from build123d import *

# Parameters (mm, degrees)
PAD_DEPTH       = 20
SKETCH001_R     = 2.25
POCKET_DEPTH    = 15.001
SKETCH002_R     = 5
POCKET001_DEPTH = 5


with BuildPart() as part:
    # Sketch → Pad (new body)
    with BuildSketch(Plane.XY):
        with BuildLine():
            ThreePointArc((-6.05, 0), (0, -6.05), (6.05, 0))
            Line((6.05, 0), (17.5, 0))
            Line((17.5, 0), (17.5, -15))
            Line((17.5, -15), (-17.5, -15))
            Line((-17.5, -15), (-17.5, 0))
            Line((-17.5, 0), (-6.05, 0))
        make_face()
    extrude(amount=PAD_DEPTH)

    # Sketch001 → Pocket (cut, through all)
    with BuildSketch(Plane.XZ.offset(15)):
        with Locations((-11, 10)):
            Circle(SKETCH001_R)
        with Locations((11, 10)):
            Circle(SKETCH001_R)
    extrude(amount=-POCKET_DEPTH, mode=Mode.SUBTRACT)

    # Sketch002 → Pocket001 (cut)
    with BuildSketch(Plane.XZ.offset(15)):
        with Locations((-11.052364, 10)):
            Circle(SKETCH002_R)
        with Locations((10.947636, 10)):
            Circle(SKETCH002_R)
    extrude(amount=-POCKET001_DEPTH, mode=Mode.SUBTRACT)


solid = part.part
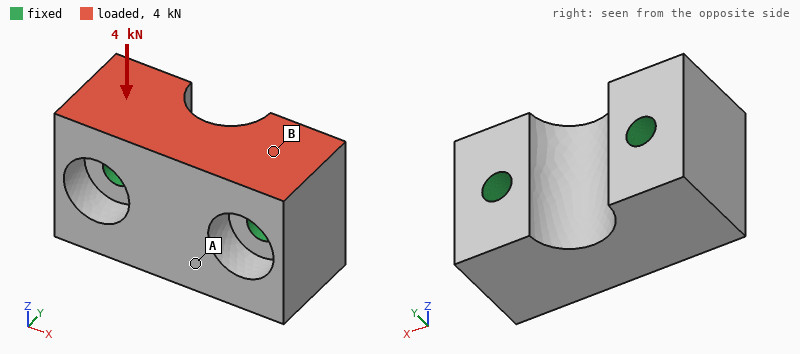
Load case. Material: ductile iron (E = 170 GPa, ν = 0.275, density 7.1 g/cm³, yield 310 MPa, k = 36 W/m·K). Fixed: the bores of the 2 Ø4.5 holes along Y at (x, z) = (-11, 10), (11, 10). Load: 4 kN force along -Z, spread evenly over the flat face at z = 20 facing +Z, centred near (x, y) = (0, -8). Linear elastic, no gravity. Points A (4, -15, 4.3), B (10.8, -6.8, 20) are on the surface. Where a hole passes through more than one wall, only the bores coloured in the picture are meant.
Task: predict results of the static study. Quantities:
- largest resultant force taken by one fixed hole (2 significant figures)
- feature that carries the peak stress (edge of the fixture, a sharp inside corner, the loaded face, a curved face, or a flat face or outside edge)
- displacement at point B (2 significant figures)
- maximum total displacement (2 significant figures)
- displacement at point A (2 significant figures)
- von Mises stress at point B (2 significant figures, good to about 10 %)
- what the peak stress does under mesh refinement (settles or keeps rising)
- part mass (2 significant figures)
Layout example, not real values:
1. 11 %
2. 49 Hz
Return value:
1. 2.0 kN
2. edge of the fixture
3. 1.3 µm
4. 2.7 µm
5. 1.6 µm
6. 16 MPa
7. keeps rising
8. 59 g
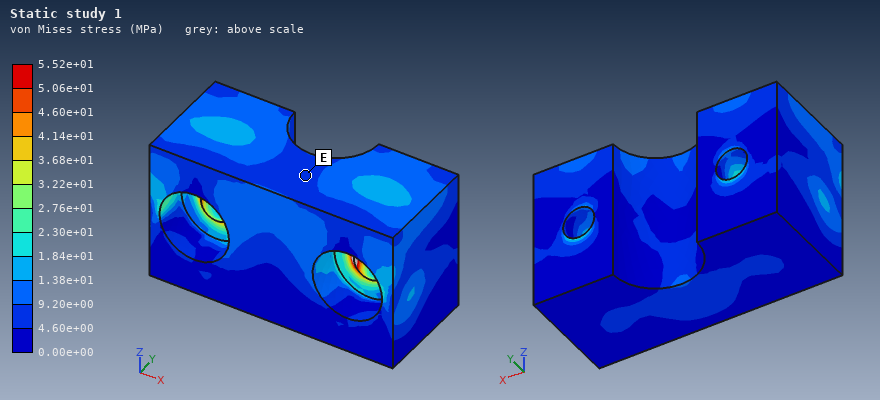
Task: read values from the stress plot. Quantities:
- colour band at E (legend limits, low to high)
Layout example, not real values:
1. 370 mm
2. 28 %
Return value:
1. 4.60e+00 to 9.20e+00 MPa
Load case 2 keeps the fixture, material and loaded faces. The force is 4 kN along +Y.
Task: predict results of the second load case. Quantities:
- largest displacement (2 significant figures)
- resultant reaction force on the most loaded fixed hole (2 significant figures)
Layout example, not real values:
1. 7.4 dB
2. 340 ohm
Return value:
1. 7.0 µm
2. 2.0 kN
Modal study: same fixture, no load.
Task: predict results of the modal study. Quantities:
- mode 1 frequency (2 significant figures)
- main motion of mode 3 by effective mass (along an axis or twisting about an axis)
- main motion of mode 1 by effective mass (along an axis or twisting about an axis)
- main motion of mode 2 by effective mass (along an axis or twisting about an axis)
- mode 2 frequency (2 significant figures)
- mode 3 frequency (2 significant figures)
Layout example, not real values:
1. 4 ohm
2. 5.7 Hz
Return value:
1. 30 kHz
2. along Y
3. along Z
4. twisting about Y
5. 41 kHz
6. 45 kHz
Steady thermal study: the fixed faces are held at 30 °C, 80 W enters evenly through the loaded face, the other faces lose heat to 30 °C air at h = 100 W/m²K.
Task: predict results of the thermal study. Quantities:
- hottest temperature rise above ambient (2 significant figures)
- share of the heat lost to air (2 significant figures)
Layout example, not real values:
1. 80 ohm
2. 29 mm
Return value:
1. 65 K
2. 7.2 %
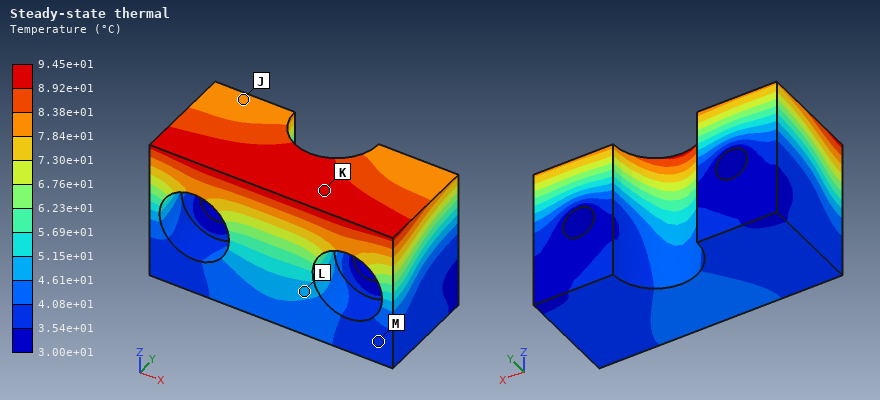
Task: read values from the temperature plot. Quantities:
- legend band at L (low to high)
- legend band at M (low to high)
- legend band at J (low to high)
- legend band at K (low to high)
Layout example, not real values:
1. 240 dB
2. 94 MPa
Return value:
1. 4.61e+01 to 5.15e+01 °C
2. 3.54e+01 to 4.08e+01 °C
3. 7.84e+01 to 8.38e+01 °C
4. 8.92e+01 to 9.45e+01 °C
